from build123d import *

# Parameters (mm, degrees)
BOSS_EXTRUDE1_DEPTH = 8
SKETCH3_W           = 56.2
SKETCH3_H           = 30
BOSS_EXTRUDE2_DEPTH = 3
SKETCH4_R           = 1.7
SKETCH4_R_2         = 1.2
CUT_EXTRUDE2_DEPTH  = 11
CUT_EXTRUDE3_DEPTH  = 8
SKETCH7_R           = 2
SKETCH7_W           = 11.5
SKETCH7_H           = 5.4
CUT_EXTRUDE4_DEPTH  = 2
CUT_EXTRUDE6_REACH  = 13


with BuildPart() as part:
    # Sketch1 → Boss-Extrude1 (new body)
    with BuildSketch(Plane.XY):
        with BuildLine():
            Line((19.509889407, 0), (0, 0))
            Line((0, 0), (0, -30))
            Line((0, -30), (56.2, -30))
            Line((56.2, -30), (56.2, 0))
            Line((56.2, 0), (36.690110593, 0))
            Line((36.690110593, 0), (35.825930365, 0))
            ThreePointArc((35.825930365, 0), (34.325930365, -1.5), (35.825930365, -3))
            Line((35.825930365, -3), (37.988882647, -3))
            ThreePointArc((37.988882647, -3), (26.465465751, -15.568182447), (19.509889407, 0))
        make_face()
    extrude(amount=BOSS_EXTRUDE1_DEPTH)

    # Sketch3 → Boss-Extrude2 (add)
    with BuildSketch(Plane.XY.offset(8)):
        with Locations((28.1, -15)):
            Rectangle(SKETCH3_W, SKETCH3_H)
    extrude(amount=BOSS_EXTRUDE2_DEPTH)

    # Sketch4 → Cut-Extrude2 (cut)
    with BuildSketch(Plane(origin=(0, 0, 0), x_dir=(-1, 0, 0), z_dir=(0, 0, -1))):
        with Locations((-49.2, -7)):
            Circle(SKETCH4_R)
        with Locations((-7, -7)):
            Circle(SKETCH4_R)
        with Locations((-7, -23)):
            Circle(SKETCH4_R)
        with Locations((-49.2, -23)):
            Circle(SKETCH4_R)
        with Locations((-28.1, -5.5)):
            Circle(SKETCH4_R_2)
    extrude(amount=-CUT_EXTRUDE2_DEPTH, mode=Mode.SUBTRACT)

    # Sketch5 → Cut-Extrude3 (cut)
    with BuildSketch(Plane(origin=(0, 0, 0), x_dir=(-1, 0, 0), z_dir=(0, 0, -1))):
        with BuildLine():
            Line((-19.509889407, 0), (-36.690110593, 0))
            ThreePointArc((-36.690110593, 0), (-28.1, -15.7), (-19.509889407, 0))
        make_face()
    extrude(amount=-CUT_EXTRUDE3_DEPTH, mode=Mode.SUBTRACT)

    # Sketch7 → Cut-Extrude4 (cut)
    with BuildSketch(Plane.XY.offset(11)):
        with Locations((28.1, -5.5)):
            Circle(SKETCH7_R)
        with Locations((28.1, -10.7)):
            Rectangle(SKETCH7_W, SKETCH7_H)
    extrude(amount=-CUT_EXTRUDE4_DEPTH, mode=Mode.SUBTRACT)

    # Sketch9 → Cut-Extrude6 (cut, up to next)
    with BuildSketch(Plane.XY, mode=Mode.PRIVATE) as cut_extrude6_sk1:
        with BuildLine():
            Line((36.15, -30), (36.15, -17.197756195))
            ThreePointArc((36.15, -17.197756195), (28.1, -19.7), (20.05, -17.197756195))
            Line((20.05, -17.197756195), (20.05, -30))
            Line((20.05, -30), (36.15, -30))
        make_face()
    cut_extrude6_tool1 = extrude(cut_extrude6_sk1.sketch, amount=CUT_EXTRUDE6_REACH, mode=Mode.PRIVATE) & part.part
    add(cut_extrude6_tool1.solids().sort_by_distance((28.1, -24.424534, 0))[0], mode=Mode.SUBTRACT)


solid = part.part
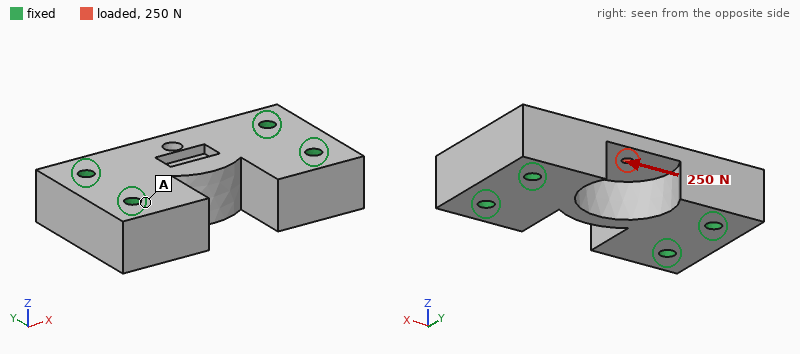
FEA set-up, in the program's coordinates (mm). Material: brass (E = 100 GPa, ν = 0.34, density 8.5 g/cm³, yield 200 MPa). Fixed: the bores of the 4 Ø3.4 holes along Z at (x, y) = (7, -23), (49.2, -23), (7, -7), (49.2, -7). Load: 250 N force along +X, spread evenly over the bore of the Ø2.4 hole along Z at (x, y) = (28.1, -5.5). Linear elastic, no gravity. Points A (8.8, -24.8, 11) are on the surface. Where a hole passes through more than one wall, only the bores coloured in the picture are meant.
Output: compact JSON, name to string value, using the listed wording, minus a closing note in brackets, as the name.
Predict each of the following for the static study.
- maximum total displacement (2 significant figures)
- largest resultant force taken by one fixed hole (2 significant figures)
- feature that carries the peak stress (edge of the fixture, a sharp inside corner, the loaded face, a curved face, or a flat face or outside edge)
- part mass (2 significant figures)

{"maximum total displacement": "1.4 µm", "largest resultant force taken by one fixed hole": "110 N", "feature that carries the peak stress": "the loaded face", "part mass": "120 g"}
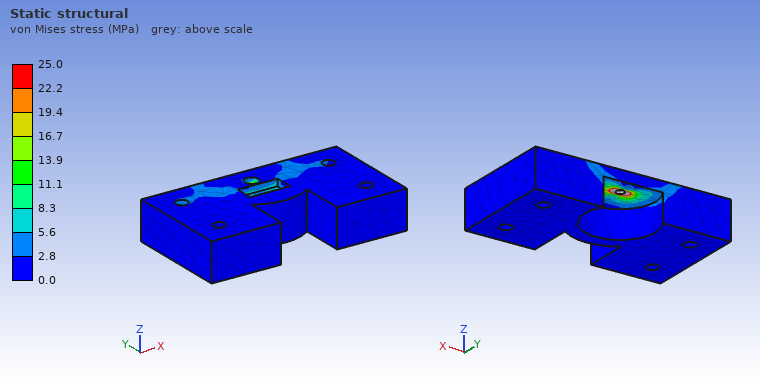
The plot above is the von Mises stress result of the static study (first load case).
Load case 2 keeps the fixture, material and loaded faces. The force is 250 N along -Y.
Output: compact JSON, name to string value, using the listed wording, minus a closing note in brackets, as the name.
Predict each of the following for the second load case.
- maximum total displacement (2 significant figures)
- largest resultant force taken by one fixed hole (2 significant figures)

{"maximum total displacement": "2.3 µm", "largest resultant force taken by one fixed hole": "120 N"}
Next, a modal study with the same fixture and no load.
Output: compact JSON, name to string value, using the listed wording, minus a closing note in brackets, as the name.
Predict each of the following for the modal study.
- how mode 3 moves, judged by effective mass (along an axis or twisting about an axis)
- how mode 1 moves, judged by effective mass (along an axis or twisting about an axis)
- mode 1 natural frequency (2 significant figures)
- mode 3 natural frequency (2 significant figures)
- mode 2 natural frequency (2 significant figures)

{"how mode 3 moves, judged by effective mass": "along Y", "how mode 1 moves, judged by effective mass": "along Z", "mode 1 natural frequency": "17 kHz", "mode 3 natural frequency": "25 kHz", "mode 2 natural frequency": "22 kHz"}
